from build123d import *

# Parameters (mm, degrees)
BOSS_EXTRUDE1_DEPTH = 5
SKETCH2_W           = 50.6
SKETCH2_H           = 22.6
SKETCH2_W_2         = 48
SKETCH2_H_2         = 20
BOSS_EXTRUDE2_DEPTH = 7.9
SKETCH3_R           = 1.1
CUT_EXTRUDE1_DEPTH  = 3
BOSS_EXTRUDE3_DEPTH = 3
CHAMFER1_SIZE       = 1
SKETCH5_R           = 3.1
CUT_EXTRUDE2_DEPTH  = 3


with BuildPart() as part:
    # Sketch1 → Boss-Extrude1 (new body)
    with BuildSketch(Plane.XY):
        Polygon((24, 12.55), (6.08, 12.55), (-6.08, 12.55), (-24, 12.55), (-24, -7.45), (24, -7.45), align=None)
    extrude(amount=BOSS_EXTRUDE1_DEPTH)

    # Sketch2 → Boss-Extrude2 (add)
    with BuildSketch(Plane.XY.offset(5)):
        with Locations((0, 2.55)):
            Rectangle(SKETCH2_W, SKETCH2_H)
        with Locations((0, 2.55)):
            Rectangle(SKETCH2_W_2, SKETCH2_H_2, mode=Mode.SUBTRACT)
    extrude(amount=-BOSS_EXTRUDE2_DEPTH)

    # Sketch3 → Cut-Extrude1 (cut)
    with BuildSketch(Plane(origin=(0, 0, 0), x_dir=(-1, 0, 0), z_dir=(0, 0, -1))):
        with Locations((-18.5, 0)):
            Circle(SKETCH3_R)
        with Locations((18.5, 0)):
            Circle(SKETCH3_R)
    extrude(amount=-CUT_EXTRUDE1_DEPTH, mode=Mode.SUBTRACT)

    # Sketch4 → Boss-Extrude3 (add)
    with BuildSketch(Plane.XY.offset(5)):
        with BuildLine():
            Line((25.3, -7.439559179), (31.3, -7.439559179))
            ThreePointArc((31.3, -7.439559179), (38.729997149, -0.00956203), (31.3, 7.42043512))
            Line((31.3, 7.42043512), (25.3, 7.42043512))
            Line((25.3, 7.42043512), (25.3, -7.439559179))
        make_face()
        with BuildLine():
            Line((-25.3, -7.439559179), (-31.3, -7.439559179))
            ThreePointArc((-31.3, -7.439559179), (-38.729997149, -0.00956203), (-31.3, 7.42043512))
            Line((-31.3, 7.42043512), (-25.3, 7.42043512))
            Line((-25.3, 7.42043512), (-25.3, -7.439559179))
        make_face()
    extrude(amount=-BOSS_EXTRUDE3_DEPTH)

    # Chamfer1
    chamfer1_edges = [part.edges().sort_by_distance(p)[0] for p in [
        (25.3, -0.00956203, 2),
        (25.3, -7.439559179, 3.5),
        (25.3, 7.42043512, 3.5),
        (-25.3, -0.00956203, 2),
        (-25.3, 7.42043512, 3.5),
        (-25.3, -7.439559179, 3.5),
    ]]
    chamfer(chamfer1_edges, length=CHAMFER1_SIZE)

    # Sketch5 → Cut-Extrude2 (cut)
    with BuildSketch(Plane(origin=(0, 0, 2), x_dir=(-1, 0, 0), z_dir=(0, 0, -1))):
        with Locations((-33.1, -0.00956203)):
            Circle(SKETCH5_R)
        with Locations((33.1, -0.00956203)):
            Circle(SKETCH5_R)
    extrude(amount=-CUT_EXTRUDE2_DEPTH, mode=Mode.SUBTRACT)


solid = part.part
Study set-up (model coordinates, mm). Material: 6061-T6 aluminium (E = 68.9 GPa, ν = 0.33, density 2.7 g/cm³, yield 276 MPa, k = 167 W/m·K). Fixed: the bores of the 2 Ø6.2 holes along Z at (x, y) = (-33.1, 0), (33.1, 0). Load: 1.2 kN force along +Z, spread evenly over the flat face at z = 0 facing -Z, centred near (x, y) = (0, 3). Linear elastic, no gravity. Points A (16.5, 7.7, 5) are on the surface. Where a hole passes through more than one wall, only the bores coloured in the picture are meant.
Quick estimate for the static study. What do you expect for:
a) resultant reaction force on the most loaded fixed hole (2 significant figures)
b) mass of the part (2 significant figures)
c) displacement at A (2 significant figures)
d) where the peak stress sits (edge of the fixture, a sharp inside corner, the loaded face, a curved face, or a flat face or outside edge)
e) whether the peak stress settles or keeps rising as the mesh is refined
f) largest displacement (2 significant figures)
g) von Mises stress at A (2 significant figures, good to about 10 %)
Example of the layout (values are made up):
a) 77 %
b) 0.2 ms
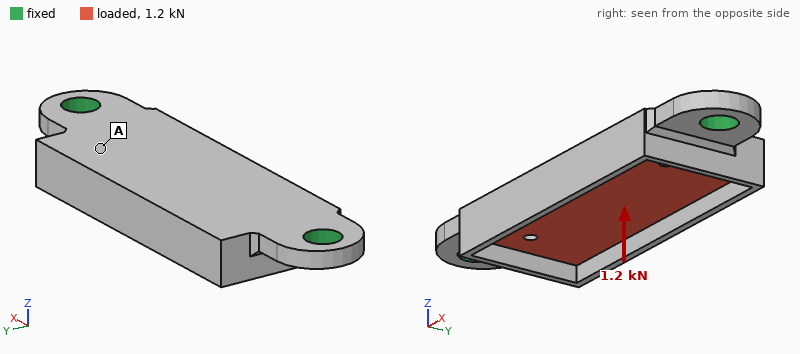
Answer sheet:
a) 1.1 kN
b) 19 g
c) 0.079 mm
d) edge of the fixture
e) keeps rising
f) 0.13 mm
g) 24 MPa
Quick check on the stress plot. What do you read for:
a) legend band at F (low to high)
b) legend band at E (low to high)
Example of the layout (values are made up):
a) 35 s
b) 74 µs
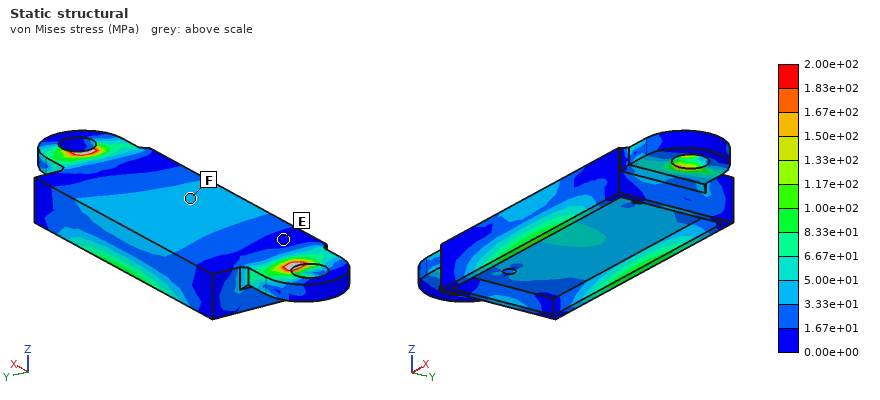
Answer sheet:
a) 3.33e+01 to 5.00e+01 MPa
b) 0.00e+00 to 1.67e+01 MPa
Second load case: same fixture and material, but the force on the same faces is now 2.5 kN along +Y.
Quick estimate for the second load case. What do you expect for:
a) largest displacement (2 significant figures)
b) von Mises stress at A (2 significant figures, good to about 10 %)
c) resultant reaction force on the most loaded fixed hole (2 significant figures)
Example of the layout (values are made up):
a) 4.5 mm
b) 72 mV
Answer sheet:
a) 0.14 mm
b) 27 MPa
c) 1.3 kN
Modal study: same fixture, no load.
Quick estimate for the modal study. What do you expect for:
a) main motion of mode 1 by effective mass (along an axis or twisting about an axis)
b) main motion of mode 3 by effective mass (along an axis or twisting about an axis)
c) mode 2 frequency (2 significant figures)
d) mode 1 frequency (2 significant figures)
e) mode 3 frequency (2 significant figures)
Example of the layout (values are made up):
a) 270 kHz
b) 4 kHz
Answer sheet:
a) along Z
b) twisting about Y
c) 6400 Hz
d) 4600 Hz
e) 12 kHz
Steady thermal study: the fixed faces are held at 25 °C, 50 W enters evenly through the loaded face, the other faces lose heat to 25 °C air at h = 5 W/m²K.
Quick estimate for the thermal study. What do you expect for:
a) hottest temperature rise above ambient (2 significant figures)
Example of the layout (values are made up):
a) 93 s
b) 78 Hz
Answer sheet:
a) 41 K
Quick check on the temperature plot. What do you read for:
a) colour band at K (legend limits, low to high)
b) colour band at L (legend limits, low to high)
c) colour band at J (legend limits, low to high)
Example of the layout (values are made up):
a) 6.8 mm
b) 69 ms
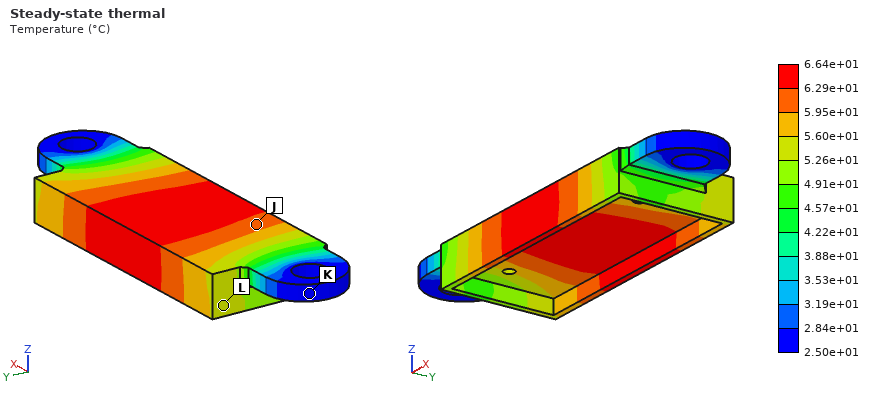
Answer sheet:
a) 2.50e+01 to 2.84e+01 °C
b) 5.26e+01 to 5.60e+01 °C
c) 5.95e+01 to 6.29e+01 °C
